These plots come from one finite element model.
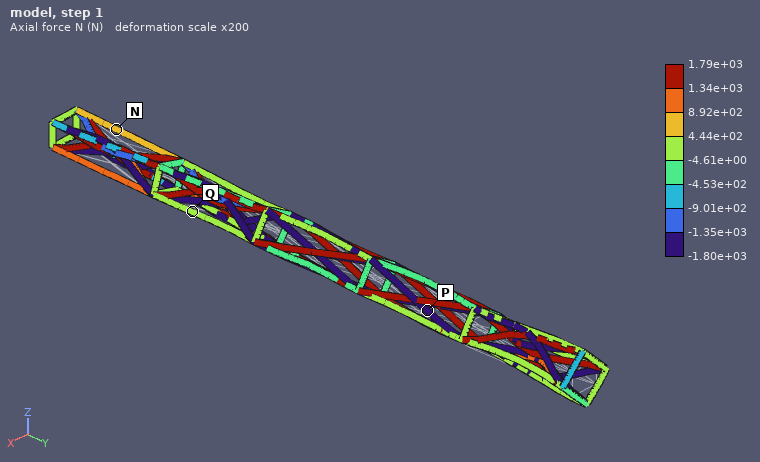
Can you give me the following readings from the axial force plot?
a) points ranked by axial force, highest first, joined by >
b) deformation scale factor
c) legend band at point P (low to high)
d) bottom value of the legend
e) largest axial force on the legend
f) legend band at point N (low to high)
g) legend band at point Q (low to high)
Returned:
N > Q > P
200
-1.80e+03 to -1.35e+03 N
-1.80e+03 N
1.79e+03 N
4.44e+02 to 8.92e+02 N
-4.61e+00 to 4.44e+02 N
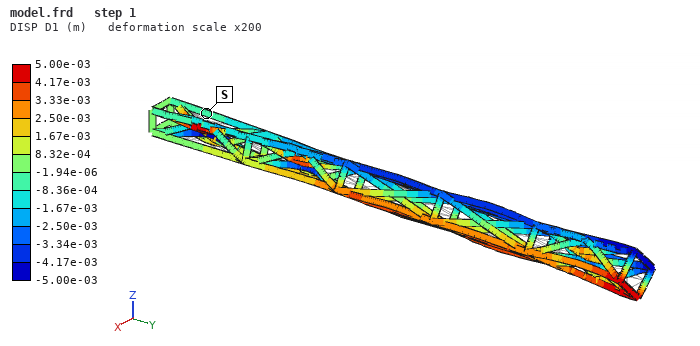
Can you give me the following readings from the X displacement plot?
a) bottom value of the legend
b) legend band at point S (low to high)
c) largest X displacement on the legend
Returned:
-5.00e-03 m
-8.36e-04 to -1.94e-06 m
5.00e-03 m
